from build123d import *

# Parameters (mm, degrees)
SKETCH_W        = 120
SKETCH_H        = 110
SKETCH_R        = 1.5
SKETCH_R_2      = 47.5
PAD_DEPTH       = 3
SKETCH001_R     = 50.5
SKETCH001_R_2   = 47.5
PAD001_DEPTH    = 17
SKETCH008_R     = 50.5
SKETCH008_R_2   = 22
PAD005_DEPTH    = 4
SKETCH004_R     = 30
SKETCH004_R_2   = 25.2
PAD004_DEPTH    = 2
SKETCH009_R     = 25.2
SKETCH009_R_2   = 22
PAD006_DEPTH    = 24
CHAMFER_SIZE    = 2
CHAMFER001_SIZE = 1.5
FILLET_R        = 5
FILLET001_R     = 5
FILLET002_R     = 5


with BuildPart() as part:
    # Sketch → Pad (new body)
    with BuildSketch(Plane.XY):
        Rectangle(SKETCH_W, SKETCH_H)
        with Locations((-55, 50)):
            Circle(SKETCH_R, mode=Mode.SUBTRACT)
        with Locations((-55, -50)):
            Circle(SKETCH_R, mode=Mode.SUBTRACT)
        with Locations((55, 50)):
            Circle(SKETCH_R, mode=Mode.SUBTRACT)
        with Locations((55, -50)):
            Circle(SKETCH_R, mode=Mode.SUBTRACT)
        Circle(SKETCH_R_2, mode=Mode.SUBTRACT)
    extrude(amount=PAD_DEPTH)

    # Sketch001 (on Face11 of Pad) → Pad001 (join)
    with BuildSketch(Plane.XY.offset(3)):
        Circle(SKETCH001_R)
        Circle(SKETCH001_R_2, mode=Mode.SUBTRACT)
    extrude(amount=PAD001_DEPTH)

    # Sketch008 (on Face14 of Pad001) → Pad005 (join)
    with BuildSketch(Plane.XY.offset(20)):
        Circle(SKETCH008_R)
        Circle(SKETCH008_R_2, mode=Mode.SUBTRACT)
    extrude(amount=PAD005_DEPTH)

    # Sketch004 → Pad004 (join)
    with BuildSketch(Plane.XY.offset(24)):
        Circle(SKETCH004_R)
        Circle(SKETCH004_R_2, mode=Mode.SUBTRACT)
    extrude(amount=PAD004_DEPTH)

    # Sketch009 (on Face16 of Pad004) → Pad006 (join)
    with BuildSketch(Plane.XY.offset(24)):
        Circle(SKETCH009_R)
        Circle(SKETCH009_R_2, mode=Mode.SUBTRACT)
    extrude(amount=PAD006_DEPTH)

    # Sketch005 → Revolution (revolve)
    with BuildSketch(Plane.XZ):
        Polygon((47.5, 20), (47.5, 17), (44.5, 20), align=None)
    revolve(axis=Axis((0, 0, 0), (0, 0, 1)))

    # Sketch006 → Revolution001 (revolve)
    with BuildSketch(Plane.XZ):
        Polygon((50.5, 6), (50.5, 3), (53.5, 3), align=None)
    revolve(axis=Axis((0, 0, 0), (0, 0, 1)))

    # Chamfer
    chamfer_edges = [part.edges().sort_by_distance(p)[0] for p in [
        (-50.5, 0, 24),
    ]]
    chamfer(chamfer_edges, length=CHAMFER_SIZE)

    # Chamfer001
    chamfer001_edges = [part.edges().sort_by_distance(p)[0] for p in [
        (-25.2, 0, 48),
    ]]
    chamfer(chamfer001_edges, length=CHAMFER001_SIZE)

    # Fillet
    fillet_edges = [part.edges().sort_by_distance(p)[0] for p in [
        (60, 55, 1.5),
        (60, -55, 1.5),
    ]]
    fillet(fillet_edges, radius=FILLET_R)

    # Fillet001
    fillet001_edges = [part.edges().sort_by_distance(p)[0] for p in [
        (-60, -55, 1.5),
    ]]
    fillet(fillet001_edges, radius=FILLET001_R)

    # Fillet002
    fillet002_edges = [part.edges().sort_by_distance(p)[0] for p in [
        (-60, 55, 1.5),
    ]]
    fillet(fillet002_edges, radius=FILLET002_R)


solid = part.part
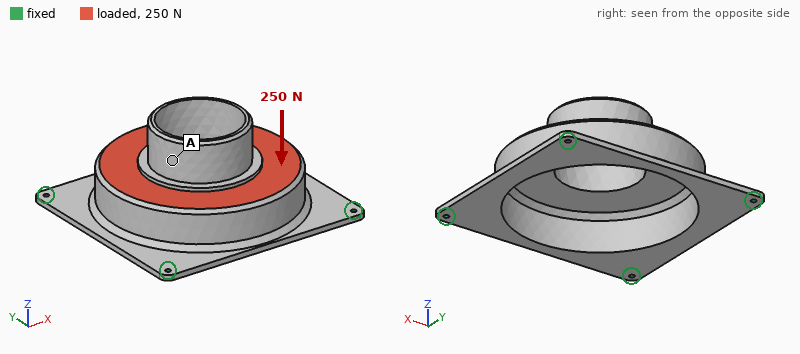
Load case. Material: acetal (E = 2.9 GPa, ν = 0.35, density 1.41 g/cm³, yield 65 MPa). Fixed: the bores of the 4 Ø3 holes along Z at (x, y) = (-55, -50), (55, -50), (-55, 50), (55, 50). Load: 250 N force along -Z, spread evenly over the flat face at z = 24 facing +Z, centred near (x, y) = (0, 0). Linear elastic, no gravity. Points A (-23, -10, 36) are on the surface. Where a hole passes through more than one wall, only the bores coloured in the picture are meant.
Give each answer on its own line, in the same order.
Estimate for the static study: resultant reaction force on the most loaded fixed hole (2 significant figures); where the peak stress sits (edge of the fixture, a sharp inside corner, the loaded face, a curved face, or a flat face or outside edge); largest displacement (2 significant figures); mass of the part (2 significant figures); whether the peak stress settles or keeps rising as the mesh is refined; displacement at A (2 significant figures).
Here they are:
91 N
edge of the fixture
0.52 mm
110 g
keeps rising
0.52 mm
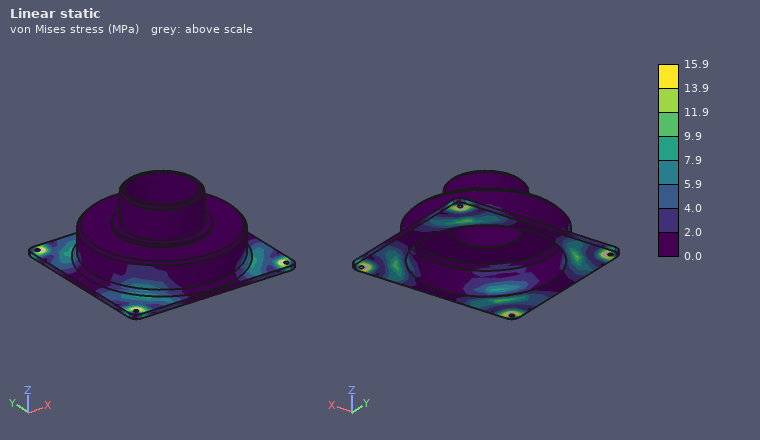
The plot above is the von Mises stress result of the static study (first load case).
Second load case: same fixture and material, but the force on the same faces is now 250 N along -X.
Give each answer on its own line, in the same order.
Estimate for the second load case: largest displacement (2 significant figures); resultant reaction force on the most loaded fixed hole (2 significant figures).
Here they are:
0.25 mm
73 N
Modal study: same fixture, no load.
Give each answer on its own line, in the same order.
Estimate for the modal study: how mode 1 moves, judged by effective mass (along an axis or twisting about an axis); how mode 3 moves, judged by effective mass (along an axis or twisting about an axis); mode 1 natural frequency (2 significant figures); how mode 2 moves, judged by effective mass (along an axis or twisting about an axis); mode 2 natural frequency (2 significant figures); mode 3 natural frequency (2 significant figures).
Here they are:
along Z
along X
360 Hz
along Y
440 Hz
470 Hz
